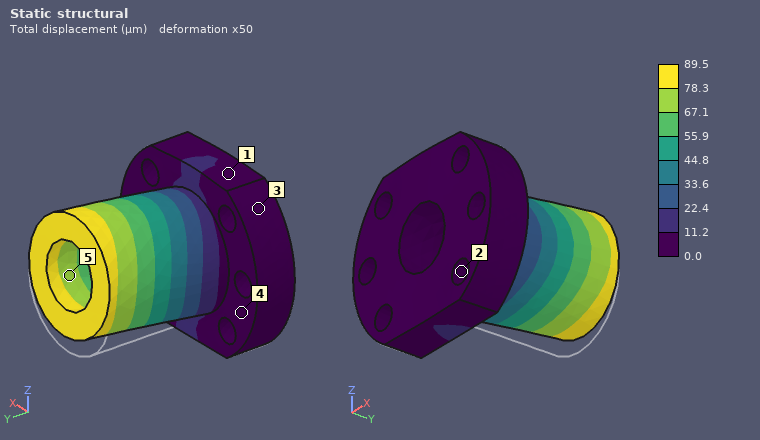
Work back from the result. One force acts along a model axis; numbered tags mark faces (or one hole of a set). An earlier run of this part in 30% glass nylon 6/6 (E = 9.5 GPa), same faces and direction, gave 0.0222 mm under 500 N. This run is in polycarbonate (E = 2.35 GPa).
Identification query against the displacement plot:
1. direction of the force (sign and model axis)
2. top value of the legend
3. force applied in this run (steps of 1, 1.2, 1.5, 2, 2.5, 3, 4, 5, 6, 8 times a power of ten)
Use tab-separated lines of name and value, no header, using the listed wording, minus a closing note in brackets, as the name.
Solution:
direction of the force	+Z
top value of the legend	89.5 µm
force applied in this run	500 N
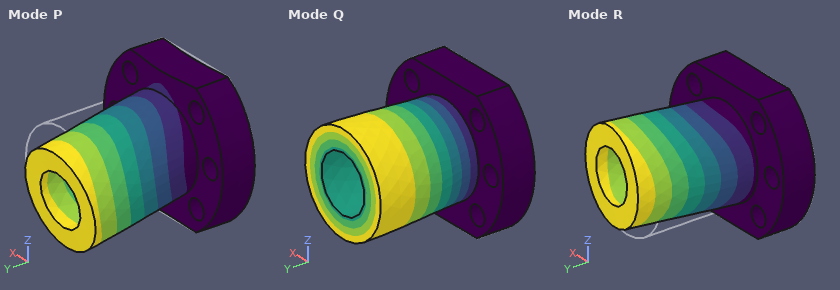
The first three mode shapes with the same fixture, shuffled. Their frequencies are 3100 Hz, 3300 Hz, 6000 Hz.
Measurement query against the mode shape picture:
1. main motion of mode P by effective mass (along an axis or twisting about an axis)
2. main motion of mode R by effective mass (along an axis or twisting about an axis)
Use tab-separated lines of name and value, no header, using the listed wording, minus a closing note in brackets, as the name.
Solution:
main motion of mode P by effective mass	along Z
main motion of mode R by effective mass	along X
